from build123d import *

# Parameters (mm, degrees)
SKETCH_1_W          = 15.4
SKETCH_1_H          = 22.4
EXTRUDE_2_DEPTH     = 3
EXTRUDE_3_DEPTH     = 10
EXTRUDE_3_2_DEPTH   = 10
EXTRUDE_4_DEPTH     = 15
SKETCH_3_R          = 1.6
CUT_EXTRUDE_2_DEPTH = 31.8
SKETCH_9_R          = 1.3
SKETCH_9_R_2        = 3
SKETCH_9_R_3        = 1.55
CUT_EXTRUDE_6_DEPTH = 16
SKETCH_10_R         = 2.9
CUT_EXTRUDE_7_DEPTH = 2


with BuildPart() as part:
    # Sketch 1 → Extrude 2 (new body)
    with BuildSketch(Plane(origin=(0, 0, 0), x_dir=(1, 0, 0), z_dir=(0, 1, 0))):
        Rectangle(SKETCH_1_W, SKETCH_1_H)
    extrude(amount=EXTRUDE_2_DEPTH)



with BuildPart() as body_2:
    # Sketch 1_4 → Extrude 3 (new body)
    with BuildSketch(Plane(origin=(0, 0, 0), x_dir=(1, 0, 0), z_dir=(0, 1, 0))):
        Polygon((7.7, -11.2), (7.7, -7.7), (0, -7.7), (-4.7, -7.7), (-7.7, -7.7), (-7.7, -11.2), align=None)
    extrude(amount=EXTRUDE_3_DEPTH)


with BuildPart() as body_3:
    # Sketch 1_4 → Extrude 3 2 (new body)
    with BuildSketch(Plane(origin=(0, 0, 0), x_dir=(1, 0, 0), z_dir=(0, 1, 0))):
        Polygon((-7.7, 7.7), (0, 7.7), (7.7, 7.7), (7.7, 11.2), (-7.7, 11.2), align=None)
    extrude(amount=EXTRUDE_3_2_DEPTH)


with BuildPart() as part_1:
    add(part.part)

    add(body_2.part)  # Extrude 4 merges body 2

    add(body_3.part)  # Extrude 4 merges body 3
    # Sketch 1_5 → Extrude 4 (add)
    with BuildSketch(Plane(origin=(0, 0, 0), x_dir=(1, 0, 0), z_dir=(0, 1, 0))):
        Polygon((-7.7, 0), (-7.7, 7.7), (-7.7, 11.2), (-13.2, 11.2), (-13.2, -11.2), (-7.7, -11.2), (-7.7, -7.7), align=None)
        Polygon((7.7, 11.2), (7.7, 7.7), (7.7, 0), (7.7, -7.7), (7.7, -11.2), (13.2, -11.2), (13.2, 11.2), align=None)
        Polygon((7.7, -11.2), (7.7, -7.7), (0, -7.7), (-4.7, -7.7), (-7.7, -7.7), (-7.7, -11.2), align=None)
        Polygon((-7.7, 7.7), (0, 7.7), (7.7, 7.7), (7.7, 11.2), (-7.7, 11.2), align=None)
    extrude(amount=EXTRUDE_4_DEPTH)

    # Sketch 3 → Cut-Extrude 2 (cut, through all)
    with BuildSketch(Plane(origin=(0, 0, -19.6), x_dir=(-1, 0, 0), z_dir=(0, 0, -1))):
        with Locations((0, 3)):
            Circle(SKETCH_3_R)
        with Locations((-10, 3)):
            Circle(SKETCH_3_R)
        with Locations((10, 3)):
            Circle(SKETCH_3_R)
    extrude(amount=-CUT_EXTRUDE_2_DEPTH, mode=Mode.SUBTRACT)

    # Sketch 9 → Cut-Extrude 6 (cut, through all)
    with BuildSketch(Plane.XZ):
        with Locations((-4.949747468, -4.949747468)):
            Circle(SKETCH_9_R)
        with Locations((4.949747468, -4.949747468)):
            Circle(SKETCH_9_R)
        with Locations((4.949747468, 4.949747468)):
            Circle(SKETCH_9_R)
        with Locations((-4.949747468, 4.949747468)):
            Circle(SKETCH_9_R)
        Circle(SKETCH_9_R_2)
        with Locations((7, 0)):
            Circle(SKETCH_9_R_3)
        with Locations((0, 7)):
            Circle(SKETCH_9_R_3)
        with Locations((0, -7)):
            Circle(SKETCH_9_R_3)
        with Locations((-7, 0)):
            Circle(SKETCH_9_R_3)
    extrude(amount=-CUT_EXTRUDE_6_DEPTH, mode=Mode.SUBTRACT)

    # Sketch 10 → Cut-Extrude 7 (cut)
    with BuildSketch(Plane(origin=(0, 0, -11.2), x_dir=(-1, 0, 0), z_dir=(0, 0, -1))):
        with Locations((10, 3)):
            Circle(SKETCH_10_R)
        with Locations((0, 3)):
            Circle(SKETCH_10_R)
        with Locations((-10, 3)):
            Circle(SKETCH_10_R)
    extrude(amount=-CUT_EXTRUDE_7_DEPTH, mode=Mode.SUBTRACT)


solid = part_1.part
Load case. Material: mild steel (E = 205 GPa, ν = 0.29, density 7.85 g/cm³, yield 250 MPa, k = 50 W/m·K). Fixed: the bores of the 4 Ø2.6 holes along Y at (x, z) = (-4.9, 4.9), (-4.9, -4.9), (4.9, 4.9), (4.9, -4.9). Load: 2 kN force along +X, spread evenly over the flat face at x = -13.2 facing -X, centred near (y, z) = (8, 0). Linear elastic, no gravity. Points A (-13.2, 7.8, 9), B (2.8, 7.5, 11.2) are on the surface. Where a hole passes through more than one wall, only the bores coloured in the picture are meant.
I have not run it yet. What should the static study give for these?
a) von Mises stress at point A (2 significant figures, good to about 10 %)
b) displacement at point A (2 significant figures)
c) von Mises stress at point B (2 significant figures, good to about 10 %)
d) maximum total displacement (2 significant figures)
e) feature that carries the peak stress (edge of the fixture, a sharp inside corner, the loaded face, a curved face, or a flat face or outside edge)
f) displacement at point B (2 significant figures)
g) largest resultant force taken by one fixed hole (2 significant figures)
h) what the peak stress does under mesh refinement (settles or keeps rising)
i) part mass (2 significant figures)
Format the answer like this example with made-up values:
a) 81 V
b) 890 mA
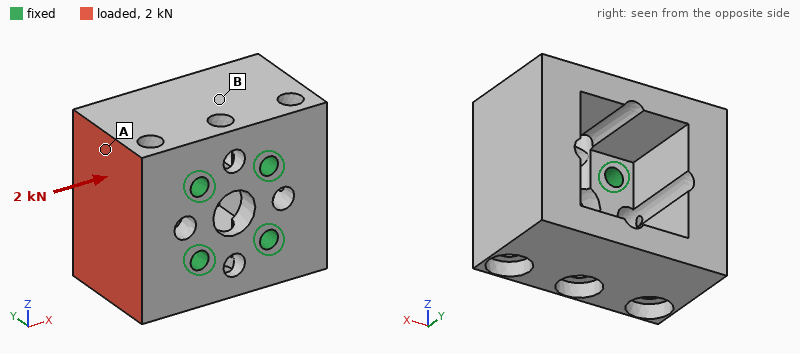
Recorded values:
a) 11 MPa
b) 6.1 µm
c) 22 MPa
d) 11 µm
e) edge of the fixture
f) 3.4 µm
g) 800 N
h) keeps rising
i) 41 g
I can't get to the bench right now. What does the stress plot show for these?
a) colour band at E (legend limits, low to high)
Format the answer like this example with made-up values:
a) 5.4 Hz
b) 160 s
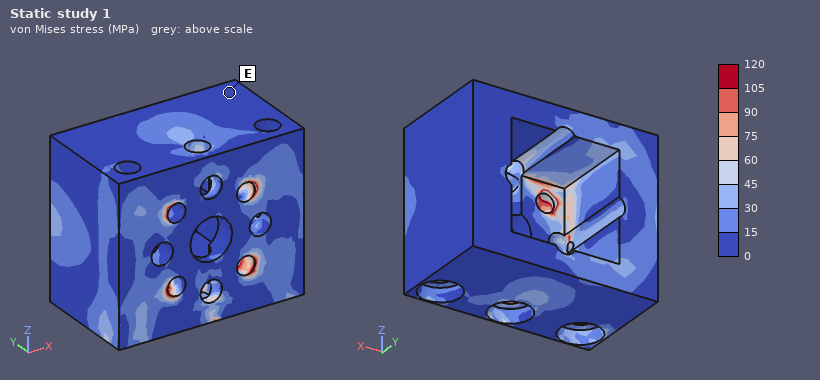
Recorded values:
a) 0 to 15 MPa
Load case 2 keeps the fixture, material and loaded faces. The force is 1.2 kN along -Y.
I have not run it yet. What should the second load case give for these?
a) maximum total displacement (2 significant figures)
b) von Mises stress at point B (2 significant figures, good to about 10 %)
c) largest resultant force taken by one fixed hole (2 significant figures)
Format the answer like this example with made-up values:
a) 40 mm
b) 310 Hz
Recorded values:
a) 9.3 µm
b) 17 MPa
c) 880 N
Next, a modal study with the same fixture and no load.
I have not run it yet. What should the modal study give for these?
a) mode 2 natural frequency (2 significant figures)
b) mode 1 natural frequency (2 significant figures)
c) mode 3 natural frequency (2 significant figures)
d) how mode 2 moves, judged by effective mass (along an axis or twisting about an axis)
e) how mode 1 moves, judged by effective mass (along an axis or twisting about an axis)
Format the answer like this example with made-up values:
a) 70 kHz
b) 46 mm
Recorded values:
a) 15 kHz
b) 14 kHz
c) 19 kHz
d) along Z
e) along X
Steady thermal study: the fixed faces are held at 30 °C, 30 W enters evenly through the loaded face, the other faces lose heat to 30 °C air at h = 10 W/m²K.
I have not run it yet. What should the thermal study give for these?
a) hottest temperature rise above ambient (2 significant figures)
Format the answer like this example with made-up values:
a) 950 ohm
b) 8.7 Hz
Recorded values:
a) 61 K
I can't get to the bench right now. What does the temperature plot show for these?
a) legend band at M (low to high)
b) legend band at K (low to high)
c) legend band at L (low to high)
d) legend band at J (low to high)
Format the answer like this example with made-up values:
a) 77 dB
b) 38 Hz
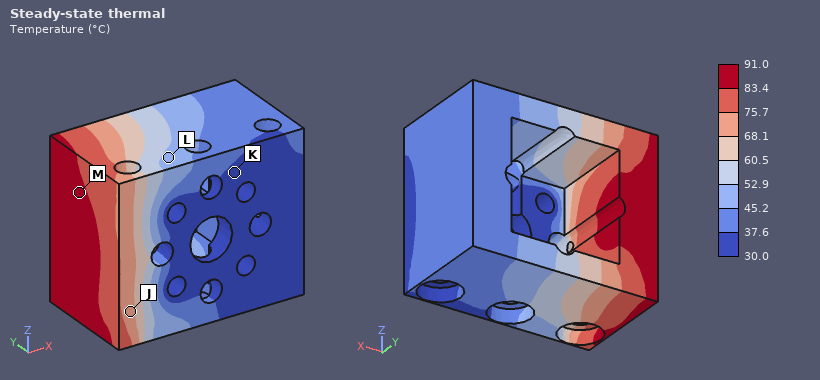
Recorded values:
a) 83.4 to 91.0 °C
b) 30.0 to 37.6 °C
c) 45.2 to 52.9 °C
d) 68.1 to 75.7 °C
